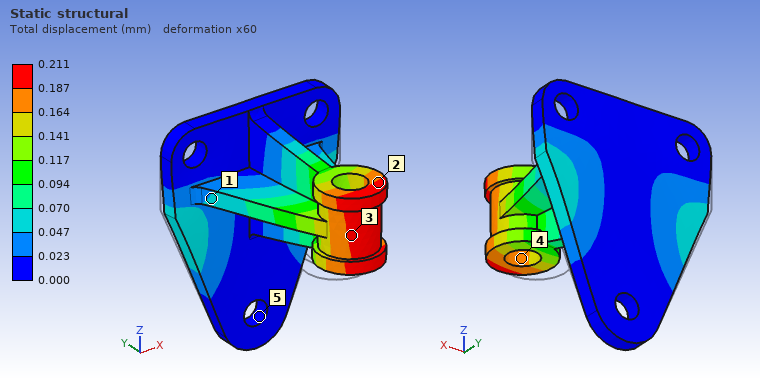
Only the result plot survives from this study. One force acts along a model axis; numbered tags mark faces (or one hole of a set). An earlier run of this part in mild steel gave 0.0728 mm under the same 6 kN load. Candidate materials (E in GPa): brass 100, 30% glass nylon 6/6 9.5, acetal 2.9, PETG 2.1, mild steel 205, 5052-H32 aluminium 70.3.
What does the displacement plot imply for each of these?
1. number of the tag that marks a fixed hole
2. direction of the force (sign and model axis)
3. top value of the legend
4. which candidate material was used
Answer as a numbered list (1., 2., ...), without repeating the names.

1. 5
2. +X
3. 0.211 mm
4. 5052-H32 aluminium
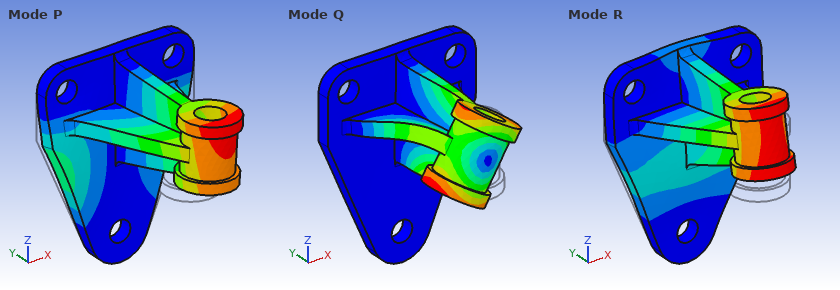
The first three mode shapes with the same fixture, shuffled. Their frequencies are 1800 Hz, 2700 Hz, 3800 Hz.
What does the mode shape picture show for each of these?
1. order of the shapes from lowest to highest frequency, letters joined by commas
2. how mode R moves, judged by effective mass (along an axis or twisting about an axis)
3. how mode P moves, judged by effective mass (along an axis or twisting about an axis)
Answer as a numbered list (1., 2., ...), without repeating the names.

1. R, P, Q
2. along Z
3. along X
